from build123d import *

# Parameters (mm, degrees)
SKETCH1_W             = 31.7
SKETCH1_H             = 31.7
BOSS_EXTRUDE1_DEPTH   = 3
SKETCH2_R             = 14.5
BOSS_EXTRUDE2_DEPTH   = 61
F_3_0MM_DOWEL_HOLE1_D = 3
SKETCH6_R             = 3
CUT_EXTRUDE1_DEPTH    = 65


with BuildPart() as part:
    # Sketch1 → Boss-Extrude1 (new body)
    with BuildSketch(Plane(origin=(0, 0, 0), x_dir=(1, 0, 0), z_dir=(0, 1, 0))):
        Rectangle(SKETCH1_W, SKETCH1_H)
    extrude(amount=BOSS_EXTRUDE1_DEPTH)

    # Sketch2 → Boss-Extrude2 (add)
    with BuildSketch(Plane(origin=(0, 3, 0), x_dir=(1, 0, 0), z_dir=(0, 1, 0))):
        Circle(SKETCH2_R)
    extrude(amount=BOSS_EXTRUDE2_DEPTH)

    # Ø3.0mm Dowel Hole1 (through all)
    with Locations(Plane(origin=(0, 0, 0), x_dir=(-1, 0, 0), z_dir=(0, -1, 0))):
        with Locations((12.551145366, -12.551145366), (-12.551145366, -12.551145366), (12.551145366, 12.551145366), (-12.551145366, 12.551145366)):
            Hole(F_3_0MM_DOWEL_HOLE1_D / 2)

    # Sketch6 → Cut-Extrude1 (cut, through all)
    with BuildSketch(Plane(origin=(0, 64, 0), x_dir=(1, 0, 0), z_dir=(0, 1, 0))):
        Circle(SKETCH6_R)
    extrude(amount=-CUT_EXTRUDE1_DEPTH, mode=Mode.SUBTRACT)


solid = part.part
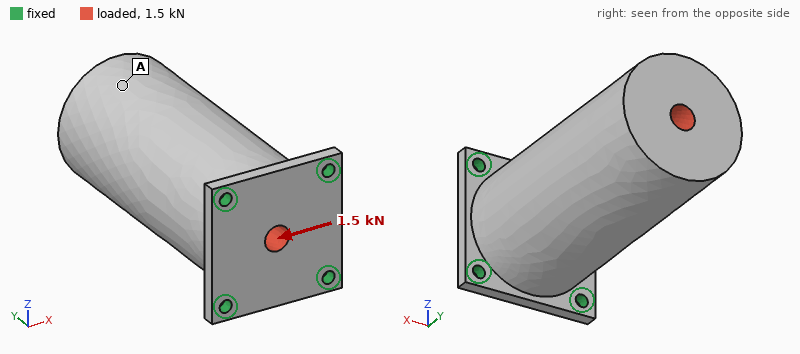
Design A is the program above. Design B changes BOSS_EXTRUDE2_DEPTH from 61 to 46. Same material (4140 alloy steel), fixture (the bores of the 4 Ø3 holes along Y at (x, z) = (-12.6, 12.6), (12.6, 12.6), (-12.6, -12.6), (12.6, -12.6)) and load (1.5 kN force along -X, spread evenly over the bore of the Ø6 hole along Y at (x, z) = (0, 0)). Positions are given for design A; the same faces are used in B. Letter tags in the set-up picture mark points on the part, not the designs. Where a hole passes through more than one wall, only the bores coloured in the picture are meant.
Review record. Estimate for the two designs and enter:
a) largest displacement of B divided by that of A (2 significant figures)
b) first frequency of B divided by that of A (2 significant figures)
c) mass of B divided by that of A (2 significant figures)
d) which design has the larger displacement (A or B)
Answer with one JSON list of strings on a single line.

["0.56", "1.5", "0.77", "A"]
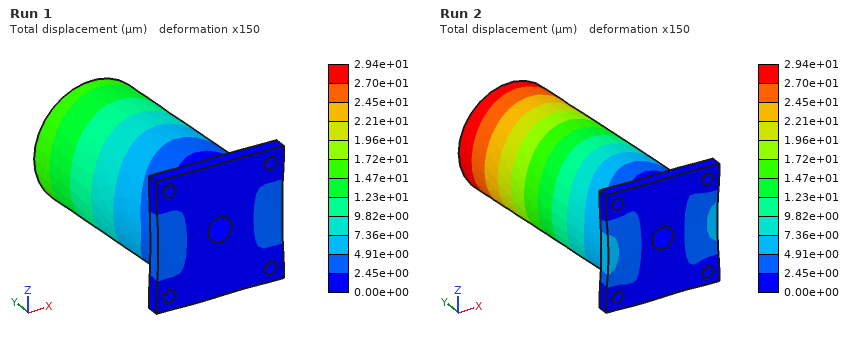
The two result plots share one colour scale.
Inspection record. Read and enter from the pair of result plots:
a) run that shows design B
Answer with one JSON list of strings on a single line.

["Run 1"]
